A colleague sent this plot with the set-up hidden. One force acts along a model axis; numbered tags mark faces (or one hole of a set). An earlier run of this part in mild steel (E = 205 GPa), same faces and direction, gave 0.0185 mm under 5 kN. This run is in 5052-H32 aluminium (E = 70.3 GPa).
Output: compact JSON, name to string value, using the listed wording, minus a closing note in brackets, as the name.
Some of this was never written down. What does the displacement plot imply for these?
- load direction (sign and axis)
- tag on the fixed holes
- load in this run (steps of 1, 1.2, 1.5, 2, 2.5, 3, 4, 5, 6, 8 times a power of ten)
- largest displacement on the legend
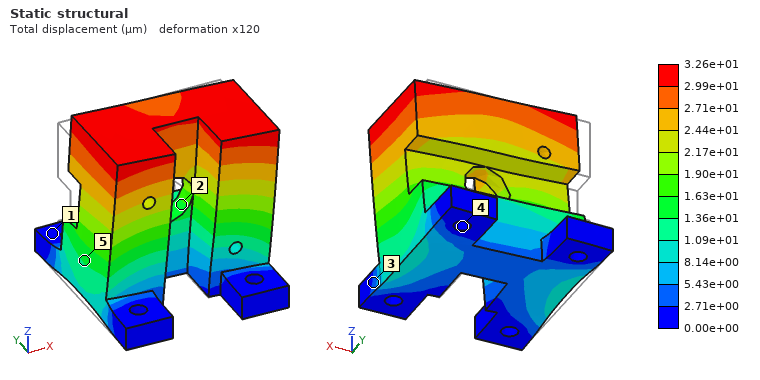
{"load direction": "+X", "tag on the fixed holes": "4", "load in this run": "3 kN", "largest displacement on the legend": "3.26e+01 µm"}
